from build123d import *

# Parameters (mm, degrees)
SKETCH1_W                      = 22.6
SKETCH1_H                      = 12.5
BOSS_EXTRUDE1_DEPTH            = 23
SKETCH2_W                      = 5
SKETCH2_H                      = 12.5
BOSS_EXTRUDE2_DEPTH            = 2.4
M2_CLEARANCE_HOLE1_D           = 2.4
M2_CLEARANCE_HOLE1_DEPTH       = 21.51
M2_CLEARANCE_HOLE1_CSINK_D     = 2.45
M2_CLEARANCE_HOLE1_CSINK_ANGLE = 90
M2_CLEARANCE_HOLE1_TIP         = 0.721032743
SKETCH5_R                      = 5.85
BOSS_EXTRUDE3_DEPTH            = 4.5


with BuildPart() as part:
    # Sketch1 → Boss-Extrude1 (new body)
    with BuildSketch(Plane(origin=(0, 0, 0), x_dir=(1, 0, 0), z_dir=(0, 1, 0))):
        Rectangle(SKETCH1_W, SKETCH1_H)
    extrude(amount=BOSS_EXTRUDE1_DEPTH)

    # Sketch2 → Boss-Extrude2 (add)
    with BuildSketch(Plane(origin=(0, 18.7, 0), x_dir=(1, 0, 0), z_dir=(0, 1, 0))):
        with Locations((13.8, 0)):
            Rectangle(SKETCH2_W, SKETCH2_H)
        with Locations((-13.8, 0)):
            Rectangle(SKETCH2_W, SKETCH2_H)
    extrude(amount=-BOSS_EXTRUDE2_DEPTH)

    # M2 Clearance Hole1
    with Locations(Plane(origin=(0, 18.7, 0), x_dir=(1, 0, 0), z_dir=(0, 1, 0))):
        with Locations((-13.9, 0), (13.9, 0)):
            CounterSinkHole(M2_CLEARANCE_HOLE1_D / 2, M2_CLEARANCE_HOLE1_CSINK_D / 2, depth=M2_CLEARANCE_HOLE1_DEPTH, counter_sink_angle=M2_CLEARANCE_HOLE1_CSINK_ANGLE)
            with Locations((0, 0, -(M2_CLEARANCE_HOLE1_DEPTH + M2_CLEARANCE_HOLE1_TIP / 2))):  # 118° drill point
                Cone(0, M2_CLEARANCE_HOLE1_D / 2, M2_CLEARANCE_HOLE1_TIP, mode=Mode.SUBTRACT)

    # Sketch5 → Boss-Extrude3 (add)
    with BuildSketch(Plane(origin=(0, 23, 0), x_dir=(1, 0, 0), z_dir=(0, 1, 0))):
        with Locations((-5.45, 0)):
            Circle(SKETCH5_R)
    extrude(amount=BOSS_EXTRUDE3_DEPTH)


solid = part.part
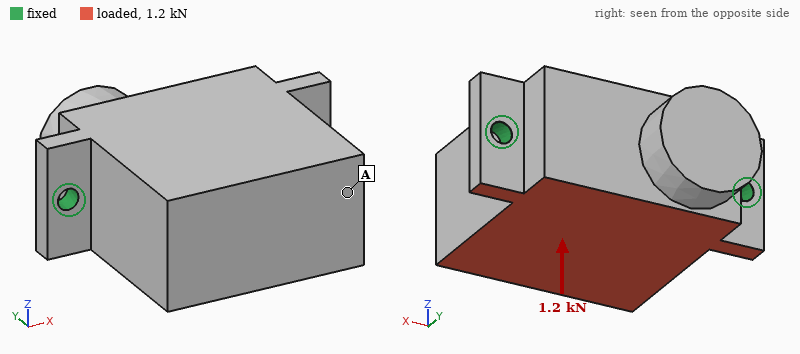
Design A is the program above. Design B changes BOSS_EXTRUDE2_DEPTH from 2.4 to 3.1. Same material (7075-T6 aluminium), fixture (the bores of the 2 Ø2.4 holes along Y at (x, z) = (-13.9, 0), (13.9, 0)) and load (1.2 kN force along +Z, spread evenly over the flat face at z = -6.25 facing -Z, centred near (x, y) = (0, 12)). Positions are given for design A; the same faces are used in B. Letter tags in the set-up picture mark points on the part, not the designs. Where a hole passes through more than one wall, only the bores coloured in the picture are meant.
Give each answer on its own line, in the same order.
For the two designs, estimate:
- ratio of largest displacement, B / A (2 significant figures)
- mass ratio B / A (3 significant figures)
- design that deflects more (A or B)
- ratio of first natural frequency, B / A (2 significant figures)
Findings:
0.56
1.01
A
1.3
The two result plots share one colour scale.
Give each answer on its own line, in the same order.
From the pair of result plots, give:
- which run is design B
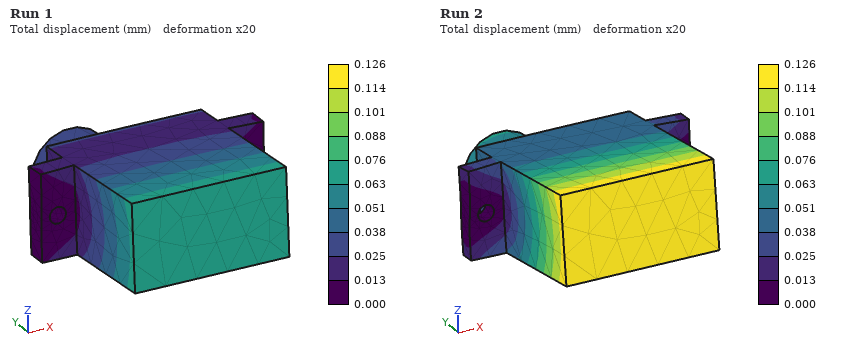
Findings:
Run 1
